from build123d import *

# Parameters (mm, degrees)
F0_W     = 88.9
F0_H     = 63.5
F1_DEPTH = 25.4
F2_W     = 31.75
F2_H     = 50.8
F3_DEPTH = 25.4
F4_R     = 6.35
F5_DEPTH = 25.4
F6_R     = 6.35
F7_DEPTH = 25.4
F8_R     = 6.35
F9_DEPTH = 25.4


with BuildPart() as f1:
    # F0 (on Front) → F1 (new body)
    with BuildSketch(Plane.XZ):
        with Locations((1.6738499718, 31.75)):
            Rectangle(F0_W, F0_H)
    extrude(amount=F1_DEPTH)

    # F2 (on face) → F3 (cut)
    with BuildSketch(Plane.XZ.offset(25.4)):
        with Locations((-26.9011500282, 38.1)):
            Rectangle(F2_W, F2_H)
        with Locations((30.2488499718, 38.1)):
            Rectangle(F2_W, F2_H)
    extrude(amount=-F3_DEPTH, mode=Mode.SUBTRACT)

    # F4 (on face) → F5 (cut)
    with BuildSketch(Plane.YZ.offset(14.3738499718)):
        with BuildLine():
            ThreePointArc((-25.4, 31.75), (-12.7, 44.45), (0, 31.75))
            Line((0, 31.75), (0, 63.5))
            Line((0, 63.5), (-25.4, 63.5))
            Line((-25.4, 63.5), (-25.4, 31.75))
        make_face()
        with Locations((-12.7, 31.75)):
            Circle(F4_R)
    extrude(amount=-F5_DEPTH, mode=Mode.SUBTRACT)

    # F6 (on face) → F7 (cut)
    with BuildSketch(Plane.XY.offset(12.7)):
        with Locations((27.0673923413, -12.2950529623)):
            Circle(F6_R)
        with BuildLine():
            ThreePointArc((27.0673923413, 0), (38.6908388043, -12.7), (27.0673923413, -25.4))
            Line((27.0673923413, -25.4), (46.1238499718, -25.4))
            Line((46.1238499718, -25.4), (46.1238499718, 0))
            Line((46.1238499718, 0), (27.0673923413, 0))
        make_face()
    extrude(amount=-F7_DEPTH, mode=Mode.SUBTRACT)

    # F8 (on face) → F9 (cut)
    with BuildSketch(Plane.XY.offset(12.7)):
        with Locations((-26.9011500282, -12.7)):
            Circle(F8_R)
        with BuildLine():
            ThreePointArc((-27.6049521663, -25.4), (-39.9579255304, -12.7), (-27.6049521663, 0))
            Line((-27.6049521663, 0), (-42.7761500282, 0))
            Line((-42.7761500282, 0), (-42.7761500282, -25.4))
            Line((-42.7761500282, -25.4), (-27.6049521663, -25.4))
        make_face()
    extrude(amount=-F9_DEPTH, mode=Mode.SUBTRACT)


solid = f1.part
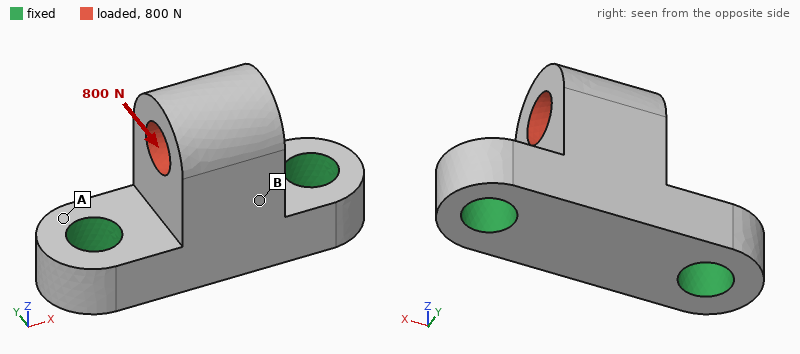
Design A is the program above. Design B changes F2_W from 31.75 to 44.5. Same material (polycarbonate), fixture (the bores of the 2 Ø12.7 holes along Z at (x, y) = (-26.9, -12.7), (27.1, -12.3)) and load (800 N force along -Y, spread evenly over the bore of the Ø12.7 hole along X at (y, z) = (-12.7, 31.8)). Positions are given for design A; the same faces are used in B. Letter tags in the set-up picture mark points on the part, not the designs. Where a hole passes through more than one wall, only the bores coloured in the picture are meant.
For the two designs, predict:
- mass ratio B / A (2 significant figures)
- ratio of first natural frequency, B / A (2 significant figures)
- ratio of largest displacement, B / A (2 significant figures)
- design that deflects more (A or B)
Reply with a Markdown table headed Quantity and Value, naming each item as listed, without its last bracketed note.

| Quantity | Value |
|---|---|
| mass ratio B / A | 0.78 |
| ratio of first natural frequency, B / A | 1.1 |
| ratio of largest displacement, B / A | 1.6 |
| design that deflects more | B |
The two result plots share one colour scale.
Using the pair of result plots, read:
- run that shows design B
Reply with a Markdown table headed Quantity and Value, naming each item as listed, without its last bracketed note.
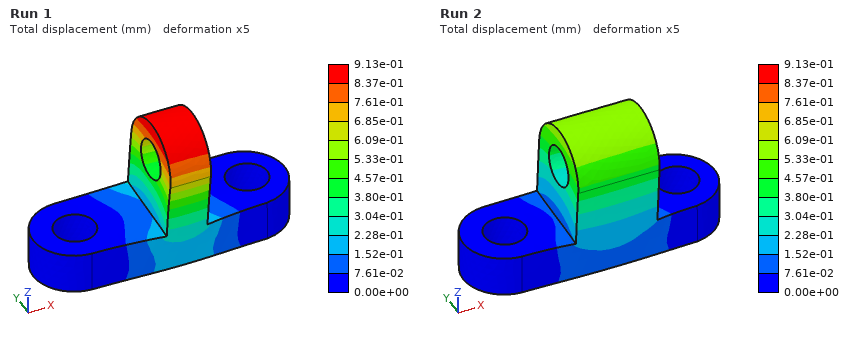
| Quantity | Value |
|---|---|
| run that shows design B | Run 1 |
